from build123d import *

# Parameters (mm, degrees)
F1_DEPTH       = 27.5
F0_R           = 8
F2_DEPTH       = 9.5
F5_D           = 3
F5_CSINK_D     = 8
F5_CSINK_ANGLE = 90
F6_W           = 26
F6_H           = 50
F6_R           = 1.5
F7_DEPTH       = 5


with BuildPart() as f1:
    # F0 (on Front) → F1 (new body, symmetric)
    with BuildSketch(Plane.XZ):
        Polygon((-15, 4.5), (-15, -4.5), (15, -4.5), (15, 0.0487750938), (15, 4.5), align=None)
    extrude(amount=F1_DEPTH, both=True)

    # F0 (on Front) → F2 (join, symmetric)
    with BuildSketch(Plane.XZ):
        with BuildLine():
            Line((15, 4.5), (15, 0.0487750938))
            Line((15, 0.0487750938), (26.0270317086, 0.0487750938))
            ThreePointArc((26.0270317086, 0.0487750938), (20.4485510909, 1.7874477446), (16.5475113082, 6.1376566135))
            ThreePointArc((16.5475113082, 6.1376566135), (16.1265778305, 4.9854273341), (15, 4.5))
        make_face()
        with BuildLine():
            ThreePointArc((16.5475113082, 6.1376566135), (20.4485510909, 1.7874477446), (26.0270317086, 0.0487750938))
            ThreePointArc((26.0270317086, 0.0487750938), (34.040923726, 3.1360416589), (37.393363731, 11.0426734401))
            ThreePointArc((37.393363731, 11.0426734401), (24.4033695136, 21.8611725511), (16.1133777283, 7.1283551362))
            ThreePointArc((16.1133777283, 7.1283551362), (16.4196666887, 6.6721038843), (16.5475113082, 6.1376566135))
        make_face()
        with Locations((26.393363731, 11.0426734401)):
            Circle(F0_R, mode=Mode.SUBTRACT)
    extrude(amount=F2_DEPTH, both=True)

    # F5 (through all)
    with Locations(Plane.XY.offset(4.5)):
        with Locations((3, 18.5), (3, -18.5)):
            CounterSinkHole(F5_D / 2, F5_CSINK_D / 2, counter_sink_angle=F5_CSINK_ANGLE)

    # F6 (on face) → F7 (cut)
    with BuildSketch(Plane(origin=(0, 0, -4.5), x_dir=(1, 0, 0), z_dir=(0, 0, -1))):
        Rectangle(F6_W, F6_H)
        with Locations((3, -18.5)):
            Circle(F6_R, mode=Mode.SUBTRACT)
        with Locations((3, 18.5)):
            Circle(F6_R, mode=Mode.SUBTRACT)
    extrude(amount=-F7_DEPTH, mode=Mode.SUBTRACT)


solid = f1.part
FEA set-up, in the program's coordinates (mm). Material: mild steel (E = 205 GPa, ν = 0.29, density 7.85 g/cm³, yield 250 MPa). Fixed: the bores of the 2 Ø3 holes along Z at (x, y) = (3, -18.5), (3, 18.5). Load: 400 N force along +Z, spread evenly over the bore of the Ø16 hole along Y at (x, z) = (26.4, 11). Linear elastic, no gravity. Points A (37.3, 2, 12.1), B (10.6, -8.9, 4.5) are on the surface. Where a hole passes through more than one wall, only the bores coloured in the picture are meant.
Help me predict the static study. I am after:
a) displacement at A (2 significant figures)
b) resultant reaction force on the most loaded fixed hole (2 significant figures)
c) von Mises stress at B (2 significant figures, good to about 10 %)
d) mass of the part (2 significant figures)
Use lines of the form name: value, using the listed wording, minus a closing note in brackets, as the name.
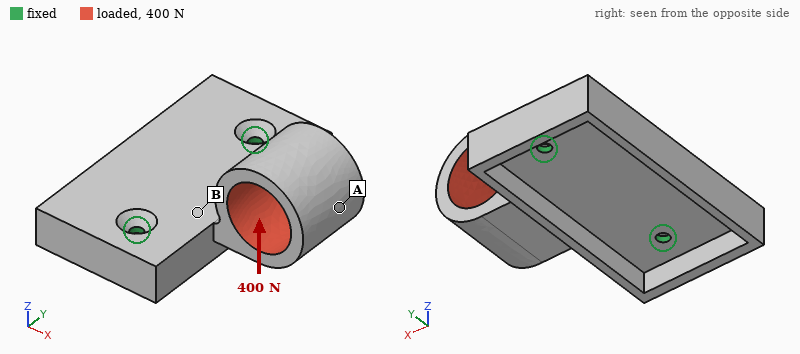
displacement at A: 0.18 mm
resultant reaction force on the most loaded fixed hole: 220 N
von Mises stress at B: 67 MPa
mass of the part: 95 g
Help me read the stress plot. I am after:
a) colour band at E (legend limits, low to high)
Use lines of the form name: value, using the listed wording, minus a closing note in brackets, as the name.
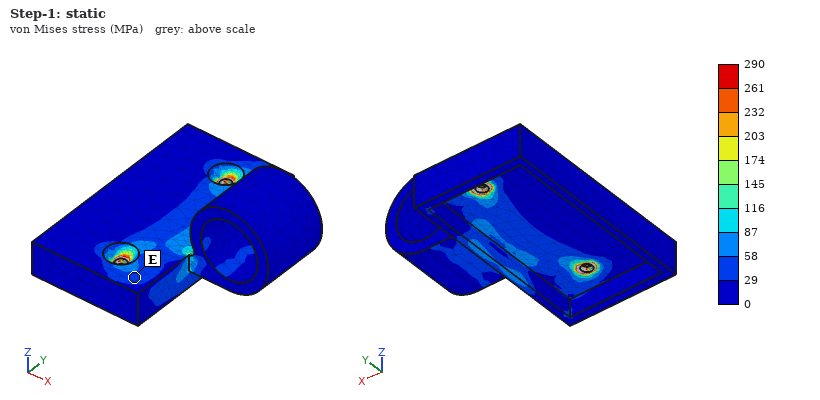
colour band at E: 29 to 58 MPa
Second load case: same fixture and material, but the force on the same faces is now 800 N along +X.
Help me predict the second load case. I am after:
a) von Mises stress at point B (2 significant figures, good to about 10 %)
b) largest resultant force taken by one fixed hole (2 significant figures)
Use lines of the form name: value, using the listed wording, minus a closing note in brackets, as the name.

von Mises stress at point B: 81 MPa
largest resultant force taken by one fixed hole: 410 N
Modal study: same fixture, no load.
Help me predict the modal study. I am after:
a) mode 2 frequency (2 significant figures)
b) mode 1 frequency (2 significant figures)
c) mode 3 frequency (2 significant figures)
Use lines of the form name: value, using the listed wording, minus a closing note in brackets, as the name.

mode 2 frequency: 4800 Hz
mode 1 frequency: 1400 Hz
mode 3 frequency: 5400 Hz
